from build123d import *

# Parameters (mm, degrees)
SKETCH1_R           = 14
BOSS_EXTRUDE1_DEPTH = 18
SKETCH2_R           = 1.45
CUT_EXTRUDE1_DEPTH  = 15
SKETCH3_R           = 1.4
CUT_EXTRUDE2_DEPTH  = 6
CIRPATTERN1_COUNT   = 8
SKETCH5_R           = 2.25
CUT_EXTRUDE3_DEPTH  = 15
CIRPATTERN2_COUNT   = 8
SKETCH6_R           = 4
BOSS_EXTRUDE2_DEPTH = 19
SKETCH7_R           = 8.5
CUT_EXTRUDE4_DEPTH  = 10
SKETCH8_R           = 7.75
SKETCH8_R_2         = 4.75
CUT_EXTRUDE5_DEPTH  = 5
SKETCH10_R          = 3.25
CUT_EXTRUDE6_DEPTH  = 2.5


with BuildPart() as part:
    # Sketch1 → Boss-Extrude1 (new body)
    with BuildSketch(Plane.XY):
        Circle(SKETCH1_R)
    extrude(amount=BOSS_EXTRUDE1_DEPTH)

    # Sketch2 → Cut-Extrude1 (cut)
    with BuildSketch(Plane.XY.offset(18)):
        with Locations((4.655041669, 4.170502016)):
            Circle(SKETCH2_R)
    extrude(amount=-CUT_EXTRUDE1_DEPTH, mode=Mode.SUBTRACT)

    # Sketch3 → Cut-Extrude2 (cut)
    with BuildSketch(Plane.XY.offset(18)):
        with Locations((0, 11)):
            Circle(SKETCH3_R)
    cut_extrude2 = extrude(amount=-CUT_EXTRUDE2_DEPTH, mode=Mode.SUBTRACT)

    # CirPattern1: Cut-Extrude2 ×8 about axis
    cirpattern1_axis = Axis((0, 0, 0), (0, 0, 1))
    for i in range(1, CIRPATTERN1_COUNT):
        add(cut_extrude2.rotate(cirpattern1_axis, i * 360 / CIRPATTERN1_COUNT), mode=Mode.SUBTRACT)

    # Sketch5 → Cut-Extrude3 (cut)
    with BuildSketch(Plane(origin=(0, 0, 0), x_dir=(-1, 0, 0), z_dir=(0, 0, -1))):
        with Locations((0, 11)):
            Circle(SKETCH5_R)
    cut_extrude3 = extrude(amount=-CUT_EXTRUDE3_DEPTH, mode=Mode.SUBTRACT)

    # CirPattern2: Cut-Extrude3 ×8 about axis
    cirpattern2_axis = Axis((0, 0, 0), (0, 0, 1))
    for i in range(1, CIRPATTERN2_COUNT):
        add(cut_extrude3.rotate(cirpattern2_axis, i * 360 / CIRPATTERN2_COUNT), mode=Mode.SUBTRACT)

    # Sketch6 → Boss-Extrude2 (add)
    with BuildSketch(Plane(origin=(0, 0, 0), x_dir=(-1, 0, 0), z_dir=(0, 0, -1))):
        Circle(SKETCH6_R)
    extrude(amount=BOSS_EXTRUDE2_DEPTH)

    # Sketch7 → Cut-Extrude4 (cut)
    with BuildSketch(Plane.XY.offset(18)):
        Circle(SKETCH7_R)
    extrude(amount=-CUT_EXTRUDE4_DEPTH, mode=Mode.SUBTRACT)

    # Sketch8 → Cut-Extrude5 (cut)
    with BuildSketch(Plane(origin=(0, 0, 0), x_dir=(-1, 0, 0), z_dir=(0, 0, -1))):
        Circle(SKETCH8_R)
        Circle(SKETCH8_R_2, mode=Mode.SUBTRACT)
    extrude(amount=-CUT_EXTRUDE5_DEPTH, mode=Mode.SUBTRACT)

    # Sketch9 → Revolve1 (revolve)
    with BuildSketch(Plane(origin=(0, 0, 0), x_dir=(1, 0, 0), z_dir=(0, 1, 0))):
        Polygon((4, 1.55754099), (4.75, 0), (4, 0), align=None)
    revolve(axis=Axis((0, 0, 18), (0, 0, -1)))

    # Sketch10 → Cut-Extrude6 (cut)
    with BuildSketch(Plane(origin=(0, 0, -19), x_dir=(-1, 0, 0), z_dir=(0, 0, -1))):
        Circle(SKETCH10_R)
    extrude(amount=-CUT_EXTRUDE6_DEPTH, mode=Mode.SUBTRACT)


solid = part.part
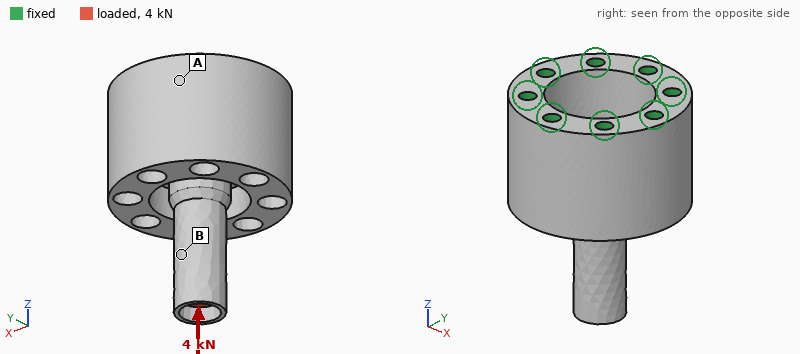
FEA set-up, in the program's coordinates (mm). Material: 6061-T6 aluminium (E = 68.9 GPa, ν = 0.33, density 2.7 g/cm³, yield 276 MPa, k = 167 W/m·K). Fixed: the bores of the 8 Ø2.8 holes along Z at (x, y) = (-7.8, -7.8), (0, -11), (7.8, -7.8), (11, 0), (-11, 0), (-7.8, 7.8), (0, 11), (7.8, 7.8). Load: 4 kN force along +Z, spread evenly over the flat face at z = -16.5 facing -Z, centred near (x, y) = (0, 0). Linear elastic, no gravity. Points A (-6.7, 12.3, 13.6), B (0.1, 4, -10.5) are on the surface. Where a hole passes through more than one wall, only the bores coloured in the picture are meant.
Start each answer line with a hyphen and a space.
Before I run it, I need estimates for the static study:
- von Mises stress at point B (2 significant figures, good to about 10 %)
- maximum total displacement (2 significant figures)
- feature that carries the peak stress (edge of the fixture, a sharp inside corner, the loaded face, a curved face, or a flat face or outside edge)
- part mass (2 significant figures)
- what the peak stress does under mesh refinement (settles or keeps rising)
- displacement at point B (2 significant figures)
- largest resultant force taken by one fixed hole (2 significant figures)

- 79 MPa
- 49 µm
- a sharp inside corner
- 19 g
- keeps rising
- 41 µm
- 540 N
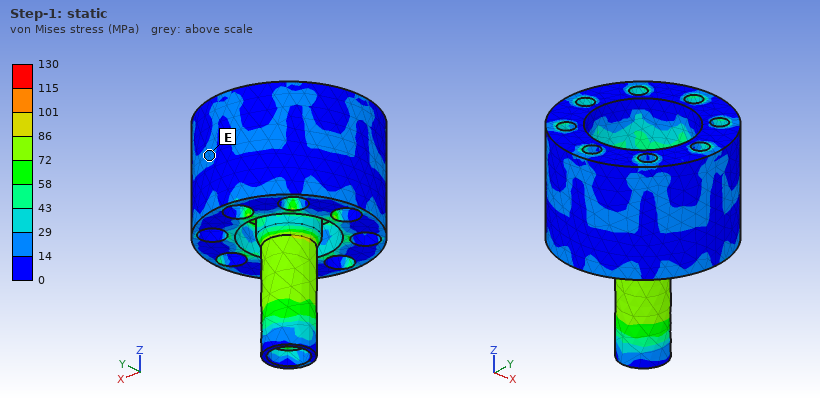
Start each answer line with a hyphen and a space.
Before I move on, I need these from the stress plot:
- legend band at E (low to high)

- 14 to 29 MPa
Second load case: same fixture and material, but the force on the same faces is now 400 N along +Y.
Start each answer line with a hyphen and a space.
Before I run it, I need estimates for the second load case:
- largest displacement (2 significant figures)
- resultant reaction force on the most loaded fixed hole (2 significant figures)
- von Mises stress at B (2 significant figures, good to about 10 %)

- 0.14 mm
- 280 N
- 48 MPa
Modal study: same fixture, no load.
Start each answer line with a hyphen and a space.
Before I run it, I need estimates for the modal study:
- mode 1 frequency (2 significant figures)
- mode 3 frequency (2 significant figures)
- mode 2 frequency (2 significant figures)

- 9200 Hz
- 22 kHz
- 9400 Hz
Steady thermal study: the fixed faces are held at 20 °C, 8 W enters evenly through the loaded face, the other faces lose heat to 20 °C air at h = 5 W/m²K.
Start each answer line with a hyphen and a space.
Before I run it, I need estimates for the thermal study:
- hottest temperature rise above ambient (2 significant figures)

- 25 K
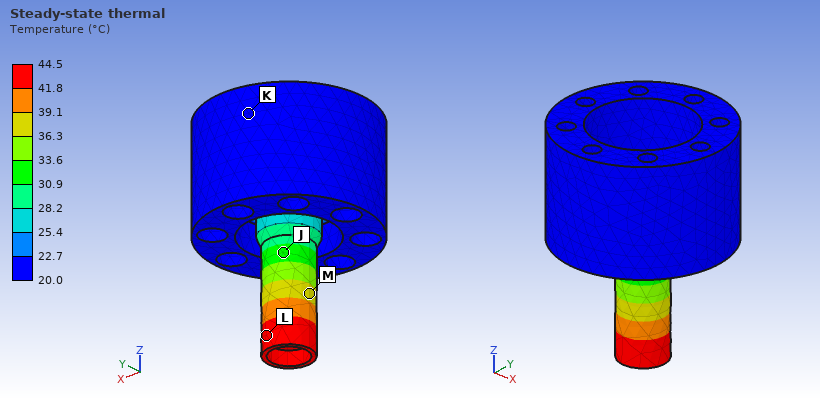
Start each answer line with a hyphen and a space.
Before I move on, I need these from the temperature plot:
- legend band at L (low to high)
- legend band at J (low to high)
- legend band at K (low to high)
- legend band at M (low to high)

- 41.8 to 44.5 °C
- 30.9 to 33.6 °C
- 20.0 to 22.7 °C
- 36.3 to 39.1 °C
